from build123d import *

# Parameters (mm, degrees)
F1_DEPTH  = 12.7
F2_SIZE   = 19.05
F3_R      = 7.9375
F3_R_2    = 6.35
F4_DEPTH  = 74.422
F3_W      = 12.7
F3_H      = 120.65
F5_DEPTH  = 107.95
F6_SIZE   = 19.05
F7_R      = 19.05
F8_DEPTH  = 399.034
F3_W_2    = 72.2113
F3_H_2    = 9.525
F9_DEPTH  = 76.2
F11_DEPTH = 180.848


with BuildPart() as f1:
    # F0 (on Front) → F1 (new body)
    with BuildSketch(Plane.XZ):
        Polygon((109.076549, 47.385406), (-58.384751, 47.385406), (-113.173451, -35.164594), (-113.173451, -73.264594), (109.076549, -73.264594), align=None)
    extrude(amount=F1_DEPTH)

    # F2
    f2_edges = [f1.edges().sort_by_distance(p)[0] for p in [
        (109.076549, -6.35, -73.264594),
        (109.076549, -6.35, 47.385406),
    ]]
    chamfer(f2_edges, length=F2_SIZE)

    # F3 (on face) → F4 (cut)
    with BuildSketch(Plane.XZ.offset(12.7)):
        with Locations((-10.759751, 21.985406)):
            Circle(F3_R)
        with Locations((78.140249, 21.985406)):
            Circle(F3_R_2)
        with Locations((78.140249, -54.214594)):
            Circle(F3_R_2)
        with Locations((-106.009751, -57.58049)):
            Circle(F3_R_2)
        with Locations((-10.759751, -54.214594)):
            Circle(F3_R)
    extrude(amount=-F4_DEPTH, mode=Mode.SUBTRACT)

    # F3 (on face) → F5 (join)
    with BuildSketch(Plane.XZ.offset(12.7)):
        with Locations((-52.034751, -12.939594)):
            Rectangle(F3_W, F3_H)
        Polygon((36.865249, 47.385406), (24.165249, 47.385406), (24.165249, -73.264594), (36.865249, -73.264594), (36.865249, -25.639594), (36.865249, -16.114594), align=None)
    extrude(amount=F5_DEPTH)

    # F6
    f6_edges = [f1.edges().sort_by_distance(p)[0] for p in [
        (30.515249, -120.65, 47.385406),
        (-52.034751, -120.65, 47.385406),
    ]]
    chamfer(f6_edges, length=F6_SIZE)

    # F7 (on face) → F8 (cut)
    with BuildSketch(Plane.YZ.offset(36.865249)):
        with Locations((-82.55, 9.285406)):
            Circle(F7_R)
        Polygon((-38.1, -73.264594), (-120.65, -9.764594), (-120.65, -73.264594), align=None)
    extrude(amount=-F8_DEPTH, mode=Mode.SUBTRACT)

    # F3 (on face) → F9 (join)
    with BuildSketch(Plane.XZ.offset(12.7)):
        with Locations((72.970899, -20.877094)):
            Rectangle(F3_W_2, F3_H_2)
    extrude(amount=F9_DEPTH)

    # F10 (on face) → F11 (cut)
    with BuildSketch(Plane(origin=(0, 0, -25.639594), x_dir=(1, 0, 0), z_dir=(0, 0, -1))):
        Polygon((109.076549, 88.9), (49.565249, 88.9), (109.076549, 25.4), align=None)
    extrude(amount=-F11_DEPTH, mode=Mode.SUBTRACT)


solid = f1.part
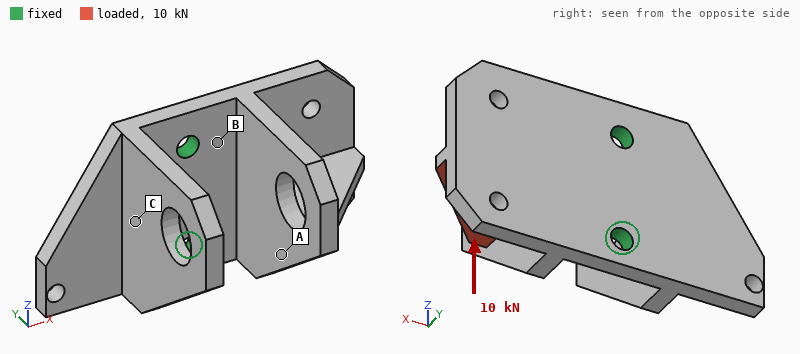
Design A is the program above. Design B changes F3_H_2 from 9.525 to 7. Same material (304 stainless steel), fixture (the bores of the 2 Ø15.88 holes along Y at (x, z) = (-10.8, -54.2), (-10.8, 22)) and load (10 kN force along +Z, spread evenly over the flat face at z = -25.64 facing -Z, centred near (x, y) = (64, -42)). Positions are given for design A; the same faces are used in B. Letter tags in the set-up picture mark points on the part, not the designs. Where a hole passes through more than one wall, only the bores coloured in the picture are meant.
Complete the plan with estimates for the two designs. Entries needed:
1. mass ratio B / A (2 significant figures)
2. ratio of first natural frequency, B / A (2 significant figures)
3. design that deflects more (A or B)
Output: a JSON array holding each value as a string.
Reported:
["0.98", "1.0", "B"]
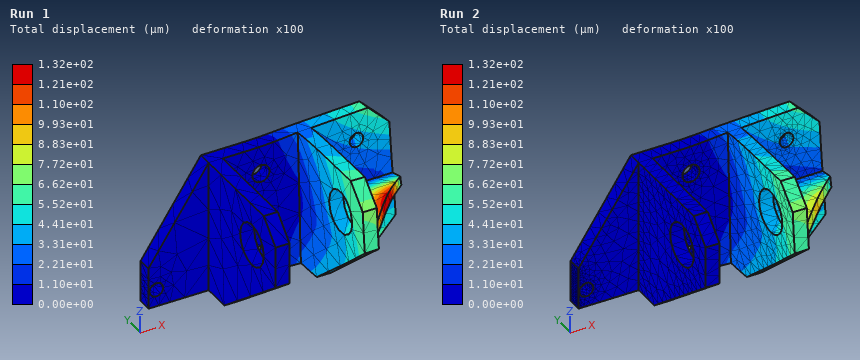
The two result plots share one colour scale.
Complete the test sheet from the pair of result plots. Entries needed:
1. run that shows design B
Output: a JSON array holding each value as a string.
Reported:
["Run 1"]
